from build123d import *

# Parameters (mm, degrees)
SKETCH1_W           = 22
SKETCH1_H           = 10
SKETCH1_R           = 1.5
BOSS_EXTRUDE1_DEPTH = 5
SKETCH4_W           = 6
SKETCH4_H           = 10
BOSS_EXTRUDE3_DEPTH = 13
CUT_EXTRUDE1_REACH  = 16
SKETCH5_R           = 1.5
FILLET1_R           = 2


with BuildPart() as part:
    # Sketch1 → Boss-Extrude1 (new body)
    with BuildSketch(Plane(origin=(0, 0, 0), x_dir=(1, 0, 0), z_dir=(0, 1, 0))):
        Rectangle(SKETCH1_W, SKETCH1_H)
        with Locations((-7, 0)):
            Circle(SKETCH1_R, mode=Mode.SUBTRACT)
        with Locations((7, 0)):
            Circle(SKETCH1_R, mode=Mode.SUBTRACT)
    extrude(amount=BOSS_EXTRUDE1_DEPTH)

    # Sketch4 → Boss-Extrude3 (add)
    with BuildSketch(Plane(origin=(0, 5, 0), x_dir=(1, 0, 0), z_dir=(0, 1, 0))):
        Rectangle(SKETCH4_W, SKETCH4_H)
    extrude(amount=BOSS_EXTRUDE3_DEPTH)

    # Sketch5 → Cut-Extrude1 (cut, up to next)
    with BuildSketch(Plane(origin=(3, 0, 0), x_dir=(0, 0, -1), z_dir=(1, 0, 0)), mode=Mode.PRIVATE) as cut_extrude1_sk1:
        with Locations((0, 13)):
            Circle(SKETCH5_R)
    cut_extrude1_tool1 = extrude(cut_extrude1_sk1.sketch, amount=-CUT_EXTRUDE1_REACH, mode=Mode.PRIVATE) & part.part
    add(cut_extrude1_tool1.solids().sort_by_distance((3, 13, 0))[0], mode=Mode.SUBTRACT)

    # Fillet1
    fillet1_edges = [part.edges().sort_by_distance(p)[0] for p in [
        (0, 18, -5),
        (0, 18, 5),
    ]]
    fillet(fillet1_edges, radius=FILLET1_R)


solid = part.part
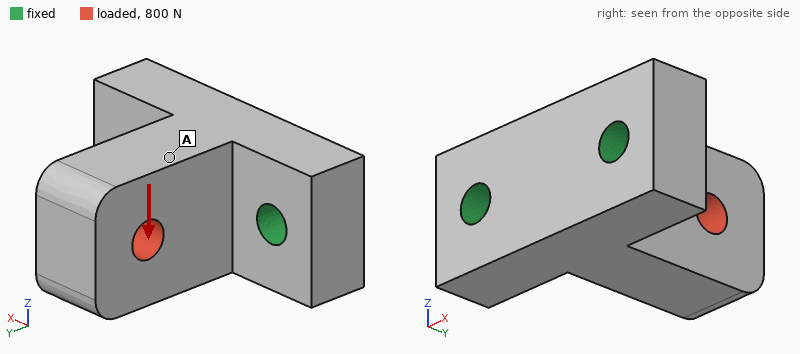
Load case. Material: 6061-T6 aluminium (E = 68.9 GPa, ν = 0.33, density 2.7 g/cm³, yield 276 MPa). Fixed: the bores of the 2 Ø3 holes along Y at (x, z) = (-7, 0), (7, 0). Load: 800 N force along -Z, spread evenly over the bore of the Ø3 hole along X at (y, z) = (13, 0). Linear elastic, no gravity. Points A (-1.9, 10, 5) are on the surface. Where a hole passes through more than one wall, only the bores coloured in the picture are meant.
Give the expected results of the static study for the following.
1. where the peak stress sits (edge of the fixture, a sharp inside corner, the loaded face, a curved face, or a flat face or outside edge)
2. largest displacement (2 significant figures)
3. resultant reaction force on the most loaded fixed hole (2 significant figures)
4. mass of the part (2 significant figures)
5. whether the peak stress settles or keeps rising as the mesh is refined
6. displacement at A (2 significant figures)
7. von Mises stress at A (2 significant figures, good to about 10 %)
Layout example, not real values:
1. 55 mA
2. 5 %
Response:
1. edge of the fixture
2. 56 µm
3. 400 N
4. 4.7 g
5. keeps rising
6. 31 µm
7. 28 MPa
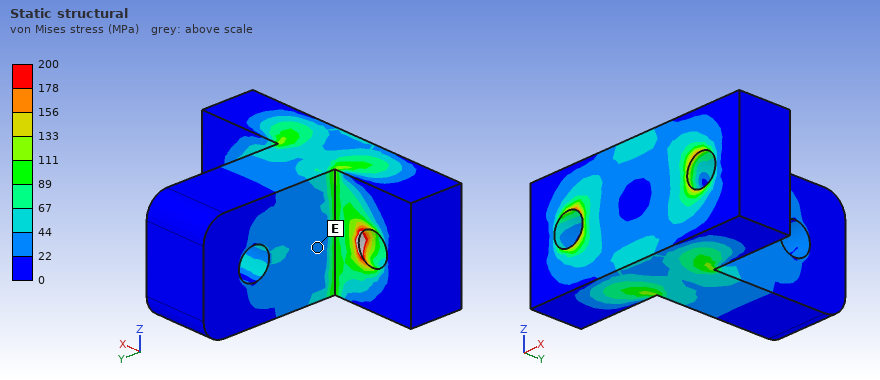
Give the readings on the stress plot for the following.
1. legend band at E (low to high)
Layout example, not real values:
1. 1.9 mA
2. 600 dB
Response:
1. 22 to 44 MPa
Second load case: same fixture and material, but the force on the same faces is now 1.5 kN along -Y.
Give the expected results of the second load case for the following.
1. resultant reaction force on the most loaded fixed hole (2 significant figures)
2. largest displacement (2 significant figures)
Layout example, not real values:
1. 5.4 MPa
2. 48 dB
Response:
1. 770 N
2. 9.5 µm
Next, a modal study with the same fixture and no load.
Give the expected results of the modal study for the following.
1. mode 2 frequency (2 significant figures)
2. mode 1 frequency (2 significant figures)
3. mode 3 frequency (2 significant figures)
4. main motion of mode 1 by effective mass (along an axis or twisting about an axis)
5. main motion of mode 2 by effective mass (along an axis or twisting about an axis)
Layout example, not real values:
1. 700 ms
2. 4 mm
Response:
1. 20 kHz
2. 17 kHz
3. 45 kHz
4. along Z
5. along X
